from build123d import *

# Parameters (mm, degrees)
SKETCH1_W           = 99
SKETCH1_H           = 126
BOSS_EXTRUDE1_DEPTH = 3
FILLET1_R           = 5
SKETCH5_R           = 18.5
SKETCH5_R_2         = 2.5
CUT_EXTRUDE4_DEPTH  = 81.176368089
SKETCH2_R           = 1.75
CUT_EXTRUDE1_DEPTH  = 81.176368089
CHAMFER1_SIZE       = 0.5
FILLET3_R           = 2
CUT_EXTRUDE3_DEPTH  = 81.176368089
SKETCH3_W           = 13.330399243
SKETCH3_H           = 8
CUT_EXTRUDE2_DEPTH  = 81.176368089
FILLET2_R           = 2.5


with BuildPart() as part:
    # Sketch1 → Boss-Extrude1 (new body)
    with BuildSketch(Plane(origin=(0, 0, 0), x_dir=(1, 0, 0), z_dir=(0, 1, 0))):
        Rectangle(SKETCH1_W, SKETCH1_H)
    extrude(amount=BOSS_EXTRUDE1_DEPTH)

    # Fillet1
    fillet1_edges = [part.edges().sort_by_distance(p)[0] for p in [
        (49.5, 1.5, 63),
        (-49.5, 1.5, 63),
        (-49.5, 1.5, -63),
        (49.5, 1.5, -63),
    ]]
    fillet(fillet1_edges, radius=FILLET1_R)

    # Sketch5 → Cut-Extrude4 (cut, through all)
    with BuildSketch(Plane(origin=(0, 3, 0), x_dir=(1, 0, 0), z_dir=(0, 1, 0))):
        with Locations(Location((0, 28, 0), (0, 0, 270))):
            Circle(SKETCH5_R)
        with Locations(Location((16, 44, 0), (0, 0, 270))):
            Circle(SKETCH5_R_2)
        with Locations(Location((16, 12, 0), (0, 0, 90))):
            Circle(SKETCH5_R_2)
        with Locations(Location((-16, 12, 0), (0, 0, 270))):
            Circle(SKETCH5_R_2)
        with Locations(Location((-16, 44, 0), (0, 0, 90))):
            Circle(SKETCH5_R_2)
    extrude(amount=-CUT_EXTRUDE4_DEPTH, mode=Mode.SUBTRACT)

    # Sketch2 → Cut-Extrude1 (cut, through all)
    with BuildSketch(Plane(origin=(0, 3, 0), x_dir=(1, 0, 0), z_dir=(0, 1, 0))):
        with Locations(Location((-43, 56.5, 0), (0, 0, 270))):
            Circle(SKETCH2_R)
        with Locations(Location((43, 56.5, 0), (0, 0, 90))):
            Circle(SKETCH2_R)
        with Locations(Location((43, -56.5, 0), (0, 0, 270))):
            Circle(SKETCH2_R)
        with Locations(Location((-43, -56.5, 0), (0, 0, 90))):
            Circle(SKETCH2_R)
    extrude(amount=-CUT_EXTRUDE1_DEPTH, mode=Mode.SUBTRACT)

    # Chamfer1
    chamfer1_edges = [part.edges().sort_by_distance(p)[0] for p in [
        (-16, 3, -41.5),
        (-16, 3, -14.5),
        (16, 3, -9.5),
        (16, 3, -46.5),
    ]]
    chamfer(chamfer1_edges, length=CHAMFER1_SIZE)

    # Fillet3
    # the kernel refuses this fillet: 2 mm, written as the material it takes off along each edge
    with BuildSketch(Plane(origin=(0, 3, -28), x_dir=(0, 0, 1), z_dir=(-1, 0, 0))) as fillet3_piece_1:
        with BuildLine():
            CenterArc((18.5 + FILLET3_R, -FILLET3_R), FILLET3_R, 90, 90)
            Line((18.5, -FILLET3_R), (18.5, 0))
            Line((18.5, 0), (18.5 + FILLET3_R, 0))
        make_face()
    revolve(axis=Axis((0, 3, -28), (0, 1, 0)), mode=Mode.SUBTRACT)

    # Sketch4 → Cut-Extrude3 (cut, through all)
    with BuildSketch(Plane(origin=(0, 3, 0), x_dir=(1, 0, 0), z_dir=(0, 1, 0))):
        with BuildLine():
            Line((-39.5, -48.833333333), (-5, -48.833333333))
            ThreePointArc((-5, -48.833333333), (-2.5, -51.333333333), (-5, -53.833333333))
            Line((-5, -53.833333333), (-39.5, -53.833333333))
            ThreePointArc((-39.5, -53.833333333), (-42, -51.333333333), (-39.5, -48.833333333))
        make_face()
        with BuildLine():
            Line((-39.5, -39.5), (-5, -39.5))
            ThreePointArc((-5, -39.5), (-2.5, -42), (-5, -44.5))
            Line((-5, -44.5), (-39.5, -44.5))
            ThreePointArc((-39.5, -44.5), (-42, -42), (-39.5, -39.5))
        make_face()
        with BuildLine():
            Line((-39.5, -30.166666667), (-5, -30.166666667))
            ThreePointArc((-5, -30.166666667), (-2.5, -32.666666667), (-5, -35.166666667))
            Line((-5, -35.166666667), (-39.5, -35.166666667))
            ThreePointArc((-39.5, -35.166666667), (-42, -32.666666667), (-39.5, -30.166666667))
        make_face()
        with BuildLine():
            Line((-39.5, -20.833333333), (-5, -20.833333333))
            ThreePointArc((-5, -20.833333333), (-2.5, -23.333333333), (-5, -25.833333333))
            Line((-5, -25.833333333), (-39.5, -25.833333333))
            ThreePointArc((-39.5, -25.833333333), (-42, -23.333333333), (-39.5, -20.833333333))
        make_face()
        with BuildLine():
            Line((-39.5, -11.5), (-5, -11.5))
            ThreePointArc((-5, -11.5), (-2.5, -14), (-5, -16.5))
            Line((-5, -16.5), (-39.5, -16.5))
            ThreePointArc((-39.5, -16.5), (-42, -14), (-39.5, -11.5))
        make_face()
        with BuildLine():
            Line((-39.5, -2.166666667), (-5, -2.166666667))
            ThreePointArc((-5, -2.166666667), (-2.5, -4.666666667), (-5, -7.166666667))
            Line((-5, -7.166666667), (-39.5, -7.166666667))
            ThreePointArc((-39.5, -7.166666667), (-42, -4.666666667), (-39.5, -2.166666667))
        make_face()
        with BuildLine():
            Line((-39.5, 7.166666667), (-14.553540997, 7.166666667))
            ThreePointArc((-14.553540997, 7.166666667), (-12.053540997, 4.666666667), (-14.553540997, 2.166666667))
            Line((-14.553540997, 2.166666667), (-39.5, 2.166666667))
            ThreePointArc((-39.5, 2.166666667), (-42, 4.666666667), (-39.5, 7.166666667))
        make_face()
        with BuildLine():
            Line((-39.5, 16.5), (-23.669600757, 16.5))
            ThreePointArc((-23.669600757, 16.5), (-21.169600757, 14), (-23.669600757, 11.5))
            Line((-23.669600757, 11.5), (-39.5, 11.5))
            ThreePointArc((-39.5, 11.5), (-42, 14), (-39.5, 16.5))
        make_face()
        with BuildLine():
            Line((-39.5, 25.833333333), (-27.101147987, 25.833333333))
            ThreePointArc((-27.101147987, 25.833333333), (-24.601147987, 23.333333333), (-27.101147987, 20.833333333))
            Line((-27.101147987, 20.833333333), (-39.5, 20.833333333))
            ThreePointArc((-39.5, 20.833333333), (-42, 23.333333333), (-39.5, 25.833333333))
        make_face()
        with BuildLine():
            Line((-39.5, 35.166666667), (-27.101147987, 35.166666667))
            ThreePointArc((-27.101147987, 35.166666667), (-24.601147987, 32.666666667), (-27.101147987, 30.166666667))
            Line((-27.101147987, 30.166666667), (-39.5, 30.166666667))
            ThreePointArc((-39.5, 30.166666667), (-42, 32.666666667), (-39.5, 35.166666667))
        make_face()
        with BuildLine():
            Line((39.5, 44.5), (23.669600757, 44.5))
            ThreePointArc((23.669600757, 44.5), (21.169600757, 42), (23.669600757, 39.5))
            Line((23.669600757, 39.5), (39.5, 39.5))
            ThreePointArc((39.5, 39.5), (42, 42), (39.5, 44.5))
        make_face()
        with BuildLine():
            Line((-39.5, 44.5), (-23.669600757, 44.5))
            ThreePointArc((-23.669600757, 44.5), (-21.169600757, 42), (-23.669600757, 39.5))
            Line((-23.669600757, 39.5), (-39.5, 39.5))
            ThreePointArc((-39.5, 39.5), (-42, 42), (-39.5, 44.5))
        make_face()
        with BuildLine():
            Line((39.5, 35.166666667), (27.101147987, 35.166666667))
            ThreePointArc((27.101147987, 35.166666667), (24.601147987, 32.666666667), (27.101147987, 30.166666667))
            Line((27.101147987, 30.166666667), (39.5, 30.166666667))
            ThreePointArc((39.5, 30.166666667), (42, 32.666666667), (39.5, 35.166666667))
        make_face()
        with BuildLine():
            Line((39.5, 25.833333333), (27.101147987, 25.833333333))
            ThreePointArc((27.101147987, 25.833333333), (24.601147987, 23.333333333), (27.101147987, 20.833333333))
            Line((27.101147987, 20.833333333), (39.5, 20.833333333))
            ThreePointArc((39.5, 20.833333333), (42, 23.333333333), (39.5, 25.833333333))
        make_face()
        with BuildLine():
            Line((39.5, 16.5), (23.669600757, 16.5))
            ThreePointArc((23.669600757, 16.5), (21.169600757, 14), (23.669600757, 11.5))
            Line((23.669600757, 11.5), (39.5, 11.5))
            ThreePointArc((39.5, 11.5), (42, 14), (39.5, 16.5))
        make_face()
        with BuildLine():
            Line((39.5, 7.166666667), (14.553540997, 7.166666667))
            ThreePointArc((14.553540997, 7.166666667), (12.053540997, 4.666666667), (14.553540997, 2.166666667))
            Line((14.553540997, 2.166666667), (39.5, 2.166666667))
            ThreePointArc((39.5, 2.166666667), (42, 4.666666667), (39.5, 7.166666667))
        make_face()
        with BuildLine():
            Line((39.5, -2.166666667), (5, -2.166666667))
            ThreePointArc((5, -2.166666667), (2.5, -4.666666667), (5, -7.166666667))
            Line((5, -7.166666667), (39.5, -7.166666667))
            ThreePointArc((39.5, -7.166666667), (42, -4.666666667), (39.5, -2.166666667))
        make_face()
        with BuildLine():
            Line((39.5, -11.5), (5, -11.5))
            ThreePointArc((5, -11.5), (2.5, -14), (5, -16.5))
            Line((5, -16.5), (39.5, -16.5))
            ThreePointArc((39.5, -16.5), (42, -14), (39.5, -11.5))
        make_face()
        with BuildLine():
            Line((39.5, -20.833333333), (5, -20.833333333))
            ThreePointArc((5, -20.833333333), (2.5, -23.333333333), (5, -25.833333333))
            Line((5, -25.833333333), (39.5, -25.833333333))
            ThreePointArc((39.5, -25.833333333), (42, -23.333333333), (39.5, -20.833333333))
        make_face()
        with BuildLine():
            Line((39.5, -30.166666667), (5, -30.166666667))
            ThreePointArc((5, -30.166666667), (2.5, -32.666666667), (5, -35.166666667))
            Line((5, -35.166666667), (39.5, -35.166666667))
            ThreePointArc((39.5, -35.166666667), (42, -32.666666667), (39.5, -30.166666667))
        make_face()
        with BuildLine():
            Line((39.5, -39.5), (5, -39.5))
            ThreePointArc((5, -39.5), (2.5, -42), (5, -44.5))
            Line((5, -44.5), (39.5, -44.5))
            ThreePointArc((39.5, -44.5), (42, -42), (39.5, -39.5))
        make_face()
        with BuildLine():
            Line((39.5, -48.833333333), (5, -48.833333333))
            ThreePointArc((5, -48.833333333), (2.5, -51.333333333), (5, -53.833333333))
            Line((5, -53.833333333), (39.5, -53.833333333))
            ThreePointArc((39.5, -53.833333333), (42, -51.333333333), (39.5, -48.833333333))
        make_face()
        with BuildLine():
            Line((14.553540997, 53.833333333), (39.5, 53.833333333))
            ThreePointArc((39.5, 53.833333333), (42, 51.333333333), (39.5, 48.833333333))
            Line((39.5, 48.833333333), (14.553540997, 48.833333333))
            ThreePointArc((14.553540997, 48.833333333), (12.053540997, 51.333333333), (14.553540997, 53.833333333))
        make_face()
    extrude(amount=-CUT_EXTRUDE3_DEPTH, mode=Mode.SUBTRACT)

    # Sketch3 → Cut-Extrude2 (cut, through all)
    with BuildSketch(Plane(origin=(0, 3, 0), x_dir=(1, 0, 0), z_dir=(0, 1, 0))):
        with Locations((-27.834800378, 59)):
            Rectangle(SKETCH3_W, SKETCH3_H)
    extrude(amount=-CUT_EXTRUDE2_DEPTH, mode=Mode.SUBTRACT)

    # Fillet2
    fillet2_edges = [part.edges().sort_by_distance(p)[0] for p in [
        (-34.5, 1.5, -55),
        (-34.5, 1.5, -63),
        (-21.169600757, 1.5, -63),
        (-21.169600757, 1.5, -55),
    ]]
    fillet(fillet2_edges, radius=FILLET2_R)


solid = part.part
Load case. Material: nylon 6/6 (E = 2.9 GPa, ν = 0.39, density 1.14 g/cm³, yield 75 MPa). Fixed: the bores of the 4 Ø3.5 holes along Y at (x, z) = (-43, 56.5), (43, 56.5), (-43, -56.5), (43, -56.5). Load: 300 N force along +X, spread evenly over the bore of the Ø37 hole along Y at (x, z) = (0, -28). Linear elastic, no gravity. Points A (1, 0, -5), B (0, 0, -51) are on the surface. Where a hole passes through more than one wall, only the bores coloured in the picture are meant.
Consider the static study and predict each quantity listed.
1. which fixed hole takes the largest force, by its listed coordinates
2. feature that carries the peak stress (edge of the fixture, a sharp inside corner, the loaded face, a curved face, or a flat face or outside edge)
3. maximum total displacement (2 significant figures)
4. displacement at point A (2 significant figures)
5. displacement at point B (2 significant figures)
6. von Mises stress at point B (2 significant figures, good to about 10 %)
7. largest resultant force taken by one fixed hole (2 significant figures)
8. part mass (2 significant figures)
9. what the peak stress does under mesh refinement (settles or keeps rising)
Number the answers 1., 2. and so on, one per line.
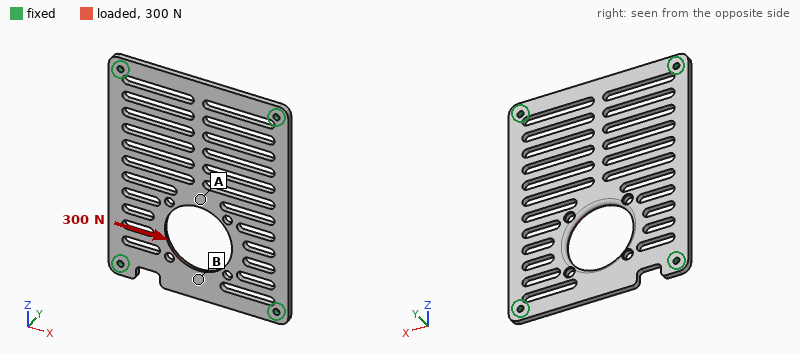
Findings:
1. (43, -56.5)
2. a sharp inside corner
3. 0.30 mm
4. 0.28 mm
5. 0.063 mm
6. 3.9 MPa
7. 160 N
8. 26 g
9. keeps rising
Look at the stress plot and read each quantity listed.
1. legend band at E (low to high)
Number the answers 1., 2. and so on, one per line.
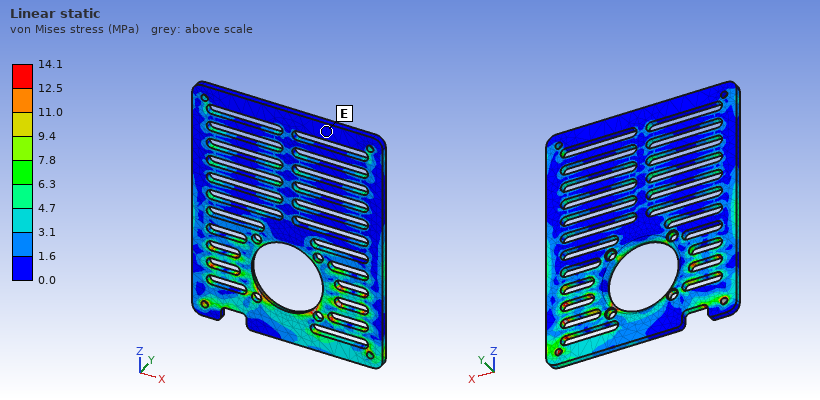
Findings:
1. 0.0 to 1.6 MPa
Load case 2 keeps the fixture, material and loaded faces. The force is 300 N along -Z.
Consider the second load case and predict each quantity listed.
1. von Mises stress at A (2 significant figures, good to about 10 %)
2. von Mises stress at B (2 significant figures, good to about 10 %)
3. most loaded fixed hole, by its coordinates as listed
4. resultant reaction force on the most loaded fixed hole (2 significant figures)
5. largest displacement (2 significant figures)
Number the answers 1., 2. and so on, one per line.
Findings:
1. 3.3 MPa
2. 1.9 MPa
3. (-43, -56.5)
4. 130 N
5. 0.42 mm
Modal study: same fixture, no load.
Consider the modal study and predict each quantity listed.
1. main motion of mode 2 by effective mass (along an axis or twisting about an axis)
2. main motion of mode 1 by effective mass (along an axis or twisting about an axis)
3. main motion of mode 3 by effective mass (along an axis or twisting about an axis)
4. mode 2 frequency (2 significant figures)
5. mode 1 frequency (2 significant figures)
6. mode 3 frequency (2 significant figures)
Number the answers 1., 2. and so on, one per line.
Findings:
1. twisting about Z
2. along Y
3. twisting about X
4. 370 Hz
5. 230 Hz
6. 530 Hz
